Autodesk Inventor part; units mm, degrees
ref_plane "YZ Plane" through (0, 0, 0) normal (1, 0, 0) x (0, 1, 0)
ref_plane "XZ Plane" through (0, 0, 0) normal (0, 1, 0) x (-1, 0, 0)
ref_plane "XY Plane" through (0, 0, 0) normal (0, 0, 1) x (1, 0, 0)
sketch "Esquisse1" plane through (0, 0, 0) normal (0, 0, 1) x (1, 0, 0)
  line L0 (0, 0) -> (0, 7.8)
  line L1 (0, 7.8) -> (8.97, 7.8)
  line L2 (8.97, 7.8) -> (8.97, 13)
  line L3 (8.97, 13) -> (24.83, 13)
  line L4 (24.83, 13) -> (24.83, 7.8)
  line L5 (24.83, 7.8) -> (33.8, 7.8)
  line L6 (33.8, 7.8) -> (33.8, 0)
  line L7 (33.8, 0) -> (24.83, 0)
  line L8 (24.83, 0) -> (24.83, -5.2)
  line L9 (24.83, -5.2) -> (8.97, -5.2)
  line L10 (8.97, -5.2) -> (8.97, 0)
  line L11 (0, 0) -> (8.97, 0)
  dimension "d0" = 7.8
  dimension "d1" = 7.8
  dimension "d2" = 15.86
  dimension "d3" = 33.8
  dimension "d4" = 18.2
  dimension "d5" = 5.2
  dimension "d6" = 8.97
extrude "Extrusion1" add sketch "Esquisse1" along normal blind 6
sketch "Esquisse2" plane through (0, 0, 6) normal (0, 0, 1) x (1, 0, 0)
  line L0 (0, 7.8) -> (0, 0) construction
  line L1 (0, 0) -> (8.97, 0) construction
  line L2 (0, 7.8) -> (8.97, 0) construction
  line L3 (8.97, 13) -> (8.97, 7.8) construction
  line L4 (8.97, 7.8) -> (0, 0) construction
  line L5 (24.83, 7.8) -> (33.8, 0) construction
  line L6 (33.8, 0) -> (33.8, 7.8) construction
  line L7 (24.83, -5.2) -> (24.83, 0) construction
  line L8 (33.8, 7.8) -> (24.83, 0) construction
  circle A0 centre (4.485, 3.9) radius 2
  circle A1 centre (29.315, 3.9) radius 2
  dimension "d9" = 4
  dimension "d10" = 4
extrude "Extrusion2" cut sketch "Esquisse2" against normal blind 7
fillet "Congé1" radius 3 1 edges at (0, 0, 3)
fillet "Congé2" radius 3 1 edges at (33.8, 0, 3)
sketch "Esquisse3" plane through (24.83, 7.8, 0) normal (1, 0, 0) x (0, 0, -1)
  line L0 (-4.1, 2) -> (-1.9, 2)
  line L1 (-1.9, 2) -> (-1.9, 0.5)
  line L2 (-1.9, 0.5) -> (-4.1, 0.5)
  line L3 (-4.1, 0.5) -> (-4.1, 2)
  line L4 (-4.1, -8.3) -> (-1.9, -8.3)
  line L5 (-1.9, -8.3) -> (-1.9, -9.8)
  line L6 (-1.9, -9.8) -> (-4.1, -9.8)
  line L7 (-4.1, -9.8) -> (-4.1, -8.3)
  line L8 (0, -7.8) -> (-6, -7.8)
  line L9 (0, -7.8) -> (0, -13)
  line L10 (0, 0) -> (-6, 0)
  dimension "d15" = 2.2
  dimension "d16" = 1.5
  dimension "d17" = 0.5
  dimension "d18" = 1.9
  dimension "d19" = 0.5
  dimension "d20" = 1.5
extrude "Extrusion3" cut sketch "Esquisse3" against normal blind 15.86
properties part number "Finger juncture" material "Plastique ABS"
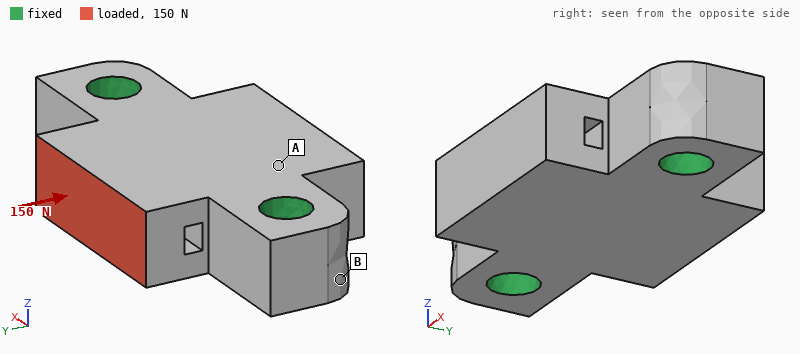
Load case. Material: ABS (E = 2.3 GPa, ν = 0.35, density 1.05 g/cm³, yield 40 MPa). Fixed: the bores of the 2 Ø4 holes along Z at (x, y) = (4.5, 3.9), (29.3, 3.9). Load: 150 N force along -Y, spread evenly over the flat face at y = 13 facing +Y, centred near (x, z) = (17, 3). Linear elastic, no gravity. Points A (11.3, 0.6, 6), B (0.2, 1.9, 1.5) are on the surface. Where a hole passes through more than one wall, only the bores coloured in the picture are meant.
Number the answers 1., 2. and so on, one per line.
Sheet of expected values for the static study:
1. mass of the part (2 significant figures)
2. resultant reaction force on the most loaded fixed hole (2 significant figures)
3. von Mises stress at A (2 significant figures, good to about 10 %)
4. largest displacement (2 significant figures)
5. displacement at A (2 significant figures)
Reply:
1. 2.4 g
2. 76 N
3. 1.4 MPa
4. 20 µm
5. 12 µm
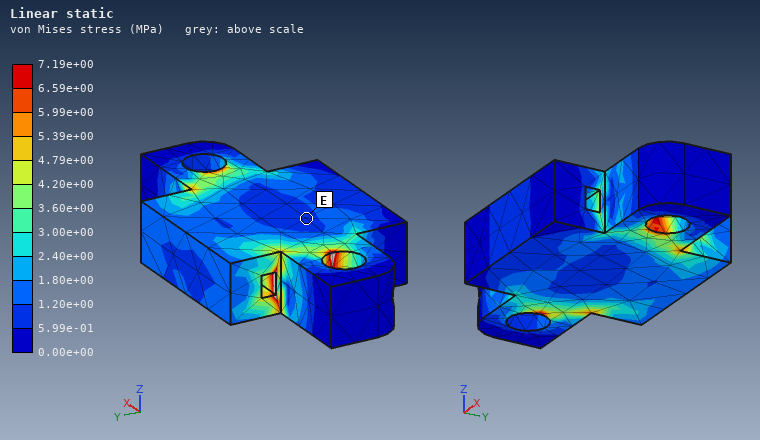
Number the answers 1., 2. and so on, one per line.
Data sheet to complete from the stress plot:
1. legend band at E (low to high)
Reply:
1. 5.99e-01 to 1.20e+00 MPa
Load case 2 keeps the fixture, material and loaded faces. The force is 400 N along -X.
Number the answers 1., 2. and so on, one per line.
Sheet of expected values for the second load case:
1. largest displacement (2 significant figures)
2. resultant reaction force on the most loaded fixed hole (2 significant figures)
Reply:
1. 0.11 mm
2. 260 N
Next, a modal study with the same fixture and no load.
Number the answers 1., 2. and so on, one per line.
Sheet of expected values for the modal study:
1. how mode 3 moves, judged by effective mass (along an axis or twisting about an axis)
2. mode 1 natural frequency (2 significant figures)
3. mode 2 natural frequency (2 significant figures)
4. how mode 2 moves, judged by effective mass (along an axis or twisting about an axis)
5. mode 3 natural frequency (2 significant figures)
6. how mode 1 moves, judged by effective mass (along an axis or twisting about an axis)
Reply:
1. along Y
2. 6900 Hz
3. 8900 Hz
4. along Z
5. 12 kHz
6. twisting about X
